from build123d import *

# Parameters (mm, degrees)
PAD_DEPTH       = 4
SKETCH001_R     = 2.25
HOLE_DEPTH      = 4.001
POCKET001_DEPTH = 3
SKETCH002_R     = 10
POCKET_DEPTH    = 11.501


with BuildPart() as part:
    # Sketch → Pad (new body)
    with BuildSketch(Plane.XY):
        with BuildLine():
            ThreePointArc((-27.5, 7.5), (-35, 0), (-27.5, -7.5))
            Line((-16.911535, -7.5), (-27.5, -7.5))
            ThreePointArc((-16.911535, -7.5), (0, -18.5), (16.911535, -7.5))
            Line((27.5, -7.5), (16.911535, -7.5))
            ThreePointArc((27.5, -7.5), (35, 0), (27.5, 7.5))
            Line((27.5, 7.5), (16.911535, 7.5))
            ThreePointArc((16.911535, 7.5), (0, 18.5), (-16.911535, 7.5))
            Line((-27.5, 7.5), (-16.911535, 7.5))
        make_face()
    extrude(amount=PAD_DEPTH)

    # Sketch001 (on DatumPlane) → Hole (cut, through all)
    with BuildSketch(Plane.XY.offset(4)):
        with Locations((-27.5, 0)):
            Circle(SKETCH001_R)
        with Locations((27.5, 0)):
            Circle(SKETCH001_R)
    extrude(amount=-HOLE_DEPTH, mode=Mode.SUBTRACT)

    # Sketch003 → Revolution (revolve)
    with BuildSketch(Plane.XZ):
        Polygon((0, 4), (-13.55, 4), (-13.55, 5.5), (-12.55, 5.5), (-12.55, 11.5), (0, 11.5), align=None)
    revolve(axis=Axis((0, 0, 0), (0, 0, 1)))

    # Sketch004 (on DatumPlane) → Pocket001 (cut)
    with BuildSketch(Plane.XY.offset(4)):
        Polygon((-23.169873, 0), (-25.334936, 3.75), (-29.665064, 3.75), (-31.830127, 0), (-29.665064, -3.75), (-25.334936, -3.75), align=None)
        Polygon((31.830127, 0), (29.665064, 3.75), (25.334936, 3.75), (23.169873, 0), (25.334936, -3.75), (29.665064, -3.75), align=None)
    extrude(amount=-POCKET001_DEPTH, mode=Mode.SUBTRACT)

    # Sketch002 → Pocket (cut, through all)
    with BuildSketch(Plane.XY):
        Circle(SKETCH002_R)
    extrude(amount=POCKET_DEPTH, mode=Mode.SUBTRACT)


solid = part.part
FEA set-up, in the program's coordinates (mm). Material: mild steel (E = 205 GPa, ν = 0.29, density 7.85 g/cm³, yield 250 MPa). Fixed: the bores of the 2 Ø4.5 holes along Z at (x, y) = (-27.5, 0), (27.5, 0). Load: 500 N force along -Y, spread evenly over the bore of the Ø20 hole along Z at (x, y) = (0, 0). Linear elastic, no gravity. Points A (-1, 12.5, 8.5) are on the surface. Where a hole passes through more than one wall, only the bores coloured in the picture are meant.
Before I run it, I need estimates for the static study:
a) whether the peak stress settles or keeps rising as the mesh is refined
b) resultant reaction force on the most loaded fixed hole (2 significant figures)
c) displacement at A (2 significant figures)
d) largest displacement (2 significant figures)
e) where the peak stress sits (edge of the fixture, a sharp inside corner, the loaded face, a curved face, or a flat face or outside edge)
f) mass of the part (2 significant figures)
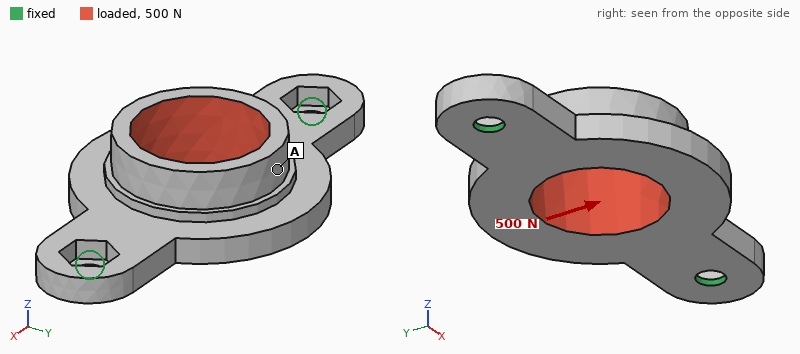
keeps rising
250 N
27 µm
33 µm
edge of the fixture
47 g
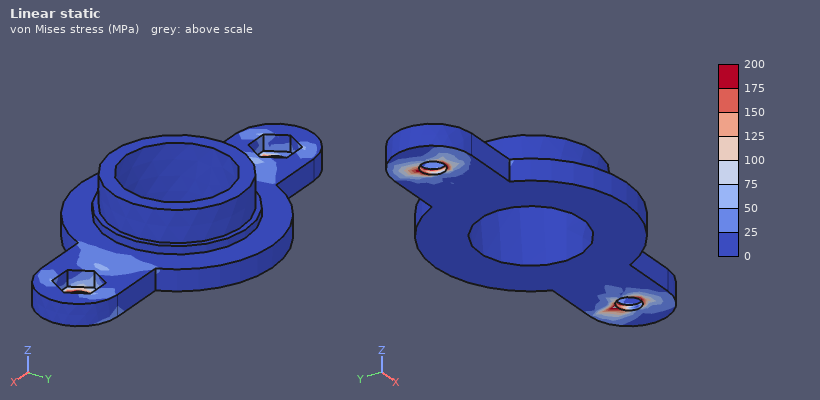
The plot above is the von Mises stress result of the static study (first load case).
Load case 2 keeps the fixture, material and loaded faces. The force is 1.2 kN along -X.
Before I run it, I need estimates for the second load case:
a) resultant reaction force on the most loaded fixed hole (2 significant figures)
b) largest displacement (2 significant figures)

610 N
3.1 µm
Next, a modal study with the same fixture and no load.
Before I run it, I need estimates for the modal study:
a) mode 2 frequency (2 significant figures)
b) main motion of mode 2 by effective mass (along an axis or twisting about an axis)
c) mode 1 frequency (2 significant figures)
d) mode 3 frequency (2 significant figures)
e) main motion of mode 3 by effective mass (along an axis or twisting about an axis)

4500 Hz
along Z
3000 Hz
11 kHz
twisting about Y
